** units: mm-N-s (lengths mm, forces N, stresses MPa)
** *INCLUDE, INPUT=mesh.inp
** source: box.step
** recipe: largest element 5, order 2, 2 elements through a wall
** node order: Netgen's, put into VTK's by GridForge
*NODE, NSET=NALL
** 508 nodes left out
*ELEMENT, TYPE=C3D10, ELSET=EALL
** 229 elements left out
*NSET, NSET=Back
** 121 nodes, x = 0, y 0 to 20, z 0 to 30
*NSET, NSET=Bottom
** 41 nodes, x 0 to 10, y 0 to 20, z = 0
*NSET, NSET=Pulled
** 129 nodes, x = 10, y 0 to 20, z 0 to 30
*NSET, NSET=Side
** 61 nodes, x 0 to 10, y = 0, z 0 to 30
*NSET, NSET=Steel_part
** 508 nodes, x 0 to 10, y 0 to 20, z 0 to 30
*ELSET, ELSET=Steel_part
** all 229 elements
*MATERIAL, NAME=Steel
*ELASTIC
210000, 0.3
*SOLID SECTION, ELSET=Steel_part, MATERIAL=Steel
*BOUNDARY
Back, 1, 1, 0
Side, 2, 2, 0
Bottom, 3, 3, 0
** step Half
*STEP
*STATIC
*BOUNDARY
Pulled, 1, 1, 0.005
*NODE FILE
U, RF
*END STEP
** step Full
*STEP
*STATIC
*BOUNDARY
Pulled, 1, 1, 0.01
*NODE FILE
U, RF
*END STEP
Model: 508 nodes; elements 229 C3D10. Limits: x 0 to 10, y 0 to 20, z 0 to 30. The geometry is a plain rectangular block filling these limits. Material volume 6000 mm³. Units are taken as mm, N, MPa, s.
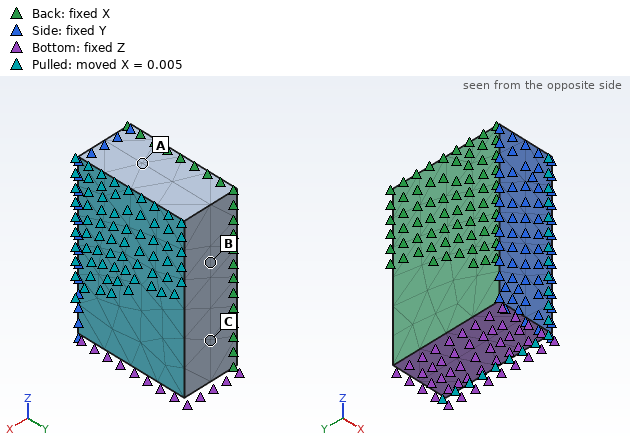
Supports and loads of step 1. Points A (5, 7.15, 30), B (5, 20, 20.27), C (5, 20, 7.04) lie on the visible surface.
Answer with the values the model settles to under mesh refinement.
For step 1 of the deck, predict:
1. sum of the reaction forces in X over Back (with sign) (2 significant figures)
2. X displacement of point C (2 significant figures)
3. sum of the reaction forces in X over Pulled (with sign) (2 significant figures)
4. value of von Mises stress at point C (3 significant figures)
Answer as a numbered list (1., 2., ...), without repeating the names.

1. -63000 N
2. 0.0025 mm
3. 63000 N
4. 105 MPa
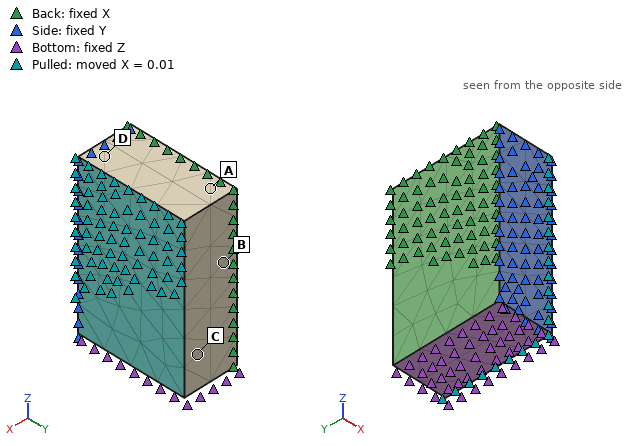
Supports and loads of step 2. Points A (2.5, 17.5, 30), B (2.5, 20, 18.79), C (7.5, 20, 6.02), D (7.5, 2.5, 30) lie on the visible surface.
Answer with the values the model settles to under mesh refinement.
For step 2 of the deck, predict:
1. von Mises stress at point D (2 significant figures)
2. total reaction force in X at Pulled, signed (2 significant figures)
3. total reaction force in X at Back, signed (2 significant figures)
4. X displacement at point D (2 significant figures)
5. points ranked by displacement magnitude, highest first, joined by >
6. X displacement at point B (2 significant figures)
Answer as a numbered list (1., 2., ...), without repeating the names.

1. 210 MPa
2. 1.3e+05 N
3. -1.3e+05 N
4. 0.0075 mm
5. D > A > C > B
6. 0.0025 mm
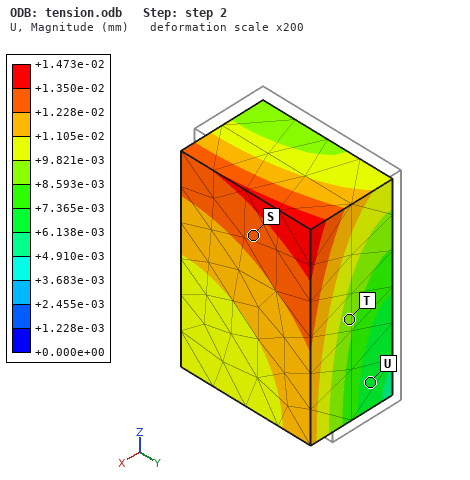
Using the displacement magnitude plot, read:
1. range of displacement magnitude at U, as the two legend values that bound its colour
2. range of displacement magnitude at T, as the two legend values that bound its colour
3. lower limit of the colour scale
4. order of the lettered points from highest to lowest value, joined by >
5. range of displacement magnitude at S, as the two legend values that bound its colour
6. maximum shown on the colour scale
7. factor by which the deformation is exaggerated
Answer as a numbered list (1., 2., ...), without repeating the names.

1. +6.138e-03 to +7.365e-03 mm
2. +8.593e-03 to +9.821e-03 mm
3. +0.000e+00 mm
4. S > T > U
5. +1.228e-02 to +1.350e-02 mm
6. +1.473e-02 mm
7. 200
